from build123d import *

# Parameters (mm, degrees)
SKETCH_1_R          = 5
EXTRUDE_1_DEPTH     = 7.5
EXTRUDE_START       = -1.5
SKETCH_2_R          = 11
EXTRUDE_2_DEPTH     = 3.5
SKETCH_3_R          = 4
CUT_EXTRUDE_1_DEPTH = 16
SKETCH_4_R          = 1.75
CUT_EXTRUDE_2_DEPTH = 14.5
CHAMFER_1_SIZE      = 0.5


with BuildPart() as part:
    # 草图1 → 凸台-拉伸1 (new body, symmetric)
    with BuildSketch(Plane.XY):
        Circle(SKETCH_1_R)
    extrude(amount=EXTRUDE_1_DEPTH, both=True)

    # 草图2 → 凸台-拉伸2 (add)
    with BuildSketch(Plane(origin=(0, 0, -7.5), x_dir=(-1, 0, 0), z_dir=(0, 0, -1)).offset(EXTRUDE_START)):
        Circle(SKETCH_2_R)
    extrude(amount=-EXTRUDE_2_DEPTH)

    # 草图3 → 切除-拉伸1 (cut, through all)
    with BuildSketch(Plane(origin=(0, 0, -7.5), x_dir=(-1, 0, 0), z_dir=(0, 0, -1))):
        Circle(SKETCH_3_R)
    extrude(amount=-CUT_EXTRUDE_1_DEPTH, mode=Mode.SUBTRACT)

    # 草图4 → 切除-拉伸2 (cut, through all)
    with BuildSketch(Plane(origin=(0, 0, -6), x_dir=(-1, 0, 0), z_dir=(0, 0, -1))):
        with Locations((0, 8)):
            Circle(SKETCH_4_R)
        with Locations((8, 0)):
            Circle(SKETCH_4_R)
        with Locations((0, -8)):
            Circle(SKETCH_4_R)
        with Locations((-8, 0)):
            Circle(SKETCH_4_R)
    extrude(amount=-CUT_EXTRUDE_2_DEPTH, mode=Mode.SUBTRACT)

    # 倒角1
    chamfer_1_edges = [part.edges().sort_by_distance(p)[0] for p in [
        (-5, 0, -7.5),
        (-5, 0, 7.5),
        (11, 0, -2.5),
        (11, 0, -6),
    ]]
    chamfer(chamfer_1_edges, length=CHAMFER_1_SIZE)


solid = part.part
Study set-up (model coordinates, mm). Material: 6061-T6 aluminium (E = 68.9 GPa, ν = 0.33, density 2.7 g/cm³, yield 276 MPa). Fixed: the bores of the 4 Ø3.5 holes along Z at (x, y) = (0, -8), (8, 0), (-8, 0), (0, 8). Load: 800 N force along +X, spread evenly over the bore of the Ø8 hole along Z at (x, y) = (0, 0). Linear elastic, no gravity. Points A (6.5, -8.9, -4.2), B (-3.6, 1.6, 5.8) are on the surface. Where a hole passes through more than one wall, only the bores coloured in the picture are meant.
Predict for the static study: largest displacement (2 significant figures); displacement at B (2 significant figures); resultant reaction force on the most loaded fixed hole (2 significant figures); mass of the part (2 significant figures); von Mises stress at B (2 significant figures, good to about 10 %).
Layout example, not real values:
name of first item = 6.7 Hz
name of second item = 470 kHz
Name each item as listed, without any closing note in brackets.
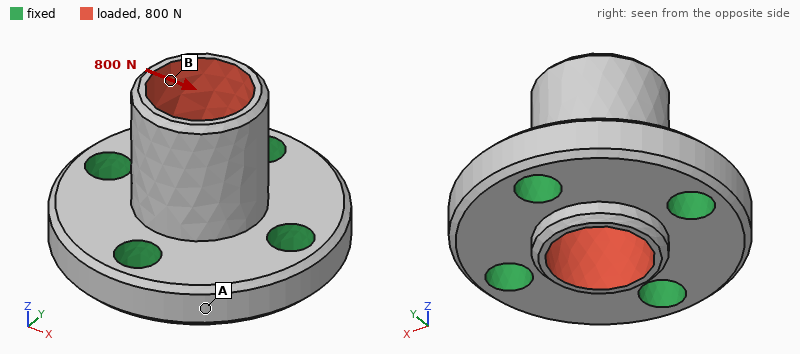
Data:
largest displacement = 15 µm
displacement at B = 13 µm
resultant reaction force on the most loaded fixed hole = 340 N
mass of the part = 3.6 g
von Mises stress at B = 11 MPa
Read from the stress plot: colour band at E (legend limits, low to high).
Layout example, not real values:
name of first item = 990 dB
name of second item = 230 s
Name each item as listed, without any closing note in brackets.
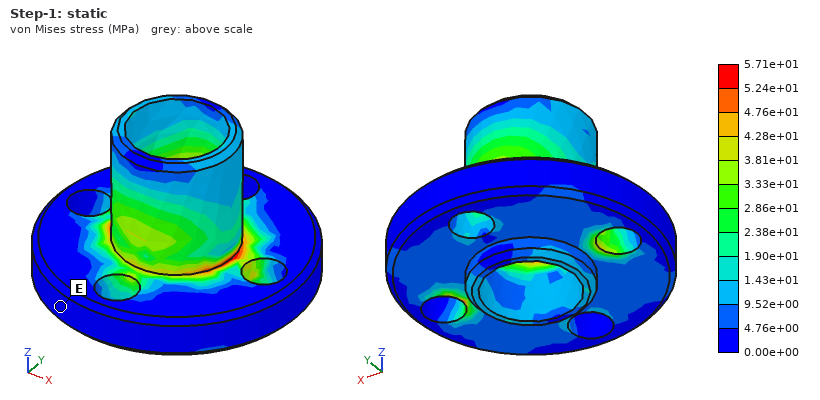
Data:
colour band at E = 0.00e+00 to 4.76e+00 MPa
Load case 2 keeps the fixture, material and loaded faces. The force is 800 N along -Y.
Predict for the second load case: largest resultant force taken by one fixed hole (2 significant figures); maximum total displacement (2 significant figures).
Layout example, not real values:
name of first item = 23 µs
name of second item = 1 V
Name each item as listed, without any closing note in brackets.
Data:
largest resultant force taken by one fixed hole = 340 N
maximum total displacement = 15 µm
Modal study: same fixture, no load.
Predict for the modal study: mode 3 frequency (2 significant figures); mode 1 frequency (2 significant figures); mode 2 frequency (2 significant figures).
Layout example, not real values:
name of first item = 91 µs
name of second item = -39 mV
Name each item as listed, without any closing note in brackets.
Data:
mode 3 frequency = 40 kHz
mode 1 frequency = 40 kHz
mode 2 frequency = 40 kHz
